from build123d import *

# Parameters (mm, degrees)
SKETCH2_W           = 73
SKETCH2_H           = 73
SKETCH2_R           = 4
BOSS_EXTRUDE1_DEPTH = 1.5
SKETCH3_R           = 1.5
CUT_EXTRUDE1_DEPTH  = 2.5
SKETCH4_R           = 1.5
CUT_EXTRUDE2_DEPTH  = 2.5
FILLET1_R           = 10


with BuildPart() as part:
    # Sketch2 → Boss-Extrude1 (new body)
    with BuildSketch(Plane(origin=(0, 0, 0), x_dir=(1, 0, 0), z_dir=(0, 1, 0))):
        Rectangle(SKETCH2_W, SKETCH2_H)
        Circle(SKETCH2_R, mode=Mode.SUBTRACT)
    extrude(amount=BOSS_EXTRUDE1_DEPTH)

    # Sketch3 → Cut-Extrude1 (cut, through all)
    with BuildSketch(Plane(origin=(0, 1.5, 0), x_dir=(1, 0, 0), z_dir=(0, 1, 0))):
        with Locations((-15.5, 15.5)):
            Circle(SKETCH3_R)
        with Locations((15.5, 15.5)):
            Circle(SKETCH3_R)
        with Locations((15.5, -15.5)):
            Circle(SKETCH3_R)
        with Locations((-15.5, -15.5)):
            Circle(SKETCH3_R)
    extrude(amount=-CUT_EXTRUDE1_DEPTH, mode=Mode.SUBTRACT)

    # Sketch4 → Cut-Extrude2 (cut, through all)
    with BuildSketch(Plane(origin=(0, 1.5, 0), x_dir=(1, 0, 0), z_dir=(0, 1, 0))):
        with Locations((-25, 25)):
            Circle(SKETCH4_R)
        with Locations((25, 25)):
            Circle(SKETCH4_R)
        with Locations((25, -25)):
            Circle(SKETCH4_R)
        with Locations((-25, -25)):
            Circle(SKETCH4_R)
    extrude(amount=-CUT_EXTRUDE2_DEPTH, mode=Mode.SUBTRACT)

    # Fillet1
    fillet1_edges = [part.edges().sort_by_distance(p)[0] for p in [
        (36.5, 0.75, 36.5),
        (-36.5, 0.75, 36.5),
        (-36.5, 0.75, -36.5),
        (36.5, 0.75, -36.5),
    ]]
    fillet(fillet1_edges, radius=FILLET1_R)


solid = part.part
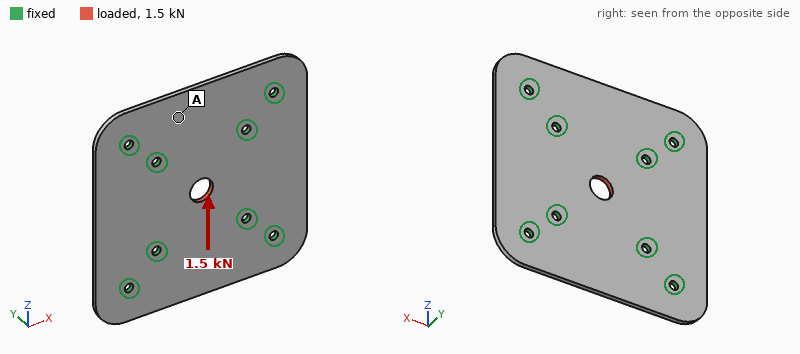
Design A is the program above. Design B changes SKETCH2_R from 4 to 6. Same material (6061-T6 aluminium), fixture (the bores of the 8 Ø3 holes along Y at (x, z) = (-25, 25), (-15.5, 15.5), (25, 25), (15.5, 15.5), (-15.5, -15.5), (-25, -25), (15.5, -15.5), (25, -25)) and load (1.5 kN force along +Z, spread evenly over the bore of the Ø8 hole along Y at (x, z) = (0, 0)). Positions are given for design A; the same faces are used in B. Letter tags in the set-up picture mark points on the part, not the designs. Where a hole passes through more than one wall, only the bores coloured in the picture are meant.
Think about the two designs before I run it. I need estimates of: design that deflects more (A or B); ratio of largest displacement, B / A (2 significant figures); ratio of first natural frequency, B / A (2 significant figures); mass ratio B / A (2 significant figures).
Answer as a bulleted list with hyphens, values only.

- A
- 0.82
- 1.0
- 0.99
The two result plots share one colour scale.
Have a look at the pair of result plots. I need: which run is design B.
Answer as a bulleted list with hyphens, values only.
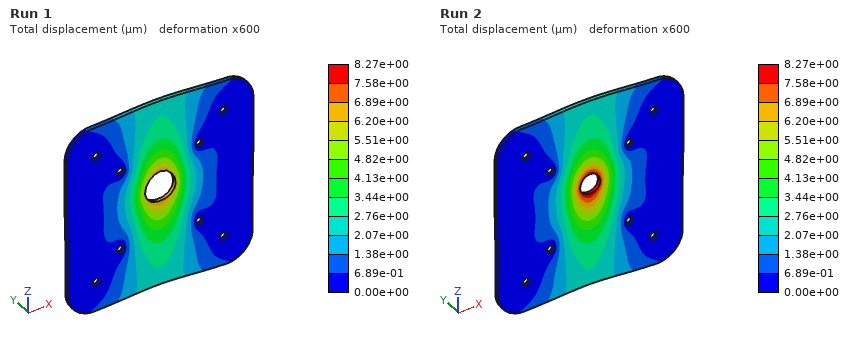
- Run 1
